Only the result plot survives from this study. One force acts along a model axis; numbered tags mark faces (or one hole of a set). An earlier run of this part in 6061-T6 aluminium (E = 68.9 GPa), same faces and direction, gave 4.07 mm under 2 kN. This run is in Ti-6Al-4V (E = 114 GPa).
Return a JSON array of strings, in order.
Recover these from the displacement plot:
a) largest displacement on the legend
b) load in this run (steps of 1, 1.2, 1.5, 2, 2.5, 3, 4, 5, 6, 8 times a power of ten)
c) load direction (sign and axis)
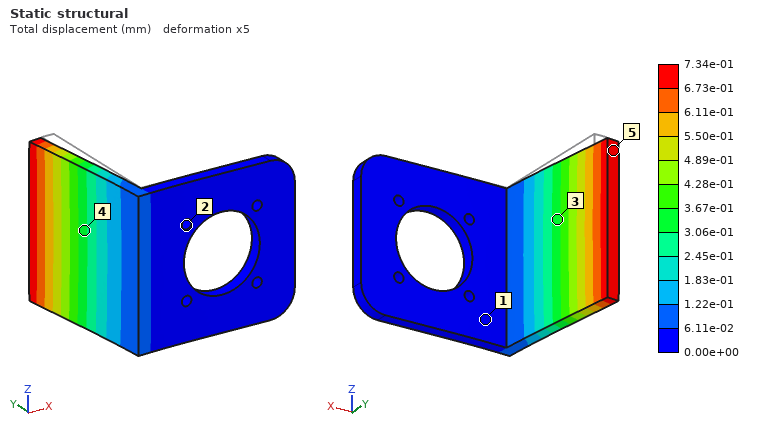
["7.34e-01 mm", "600 N", "-X"]
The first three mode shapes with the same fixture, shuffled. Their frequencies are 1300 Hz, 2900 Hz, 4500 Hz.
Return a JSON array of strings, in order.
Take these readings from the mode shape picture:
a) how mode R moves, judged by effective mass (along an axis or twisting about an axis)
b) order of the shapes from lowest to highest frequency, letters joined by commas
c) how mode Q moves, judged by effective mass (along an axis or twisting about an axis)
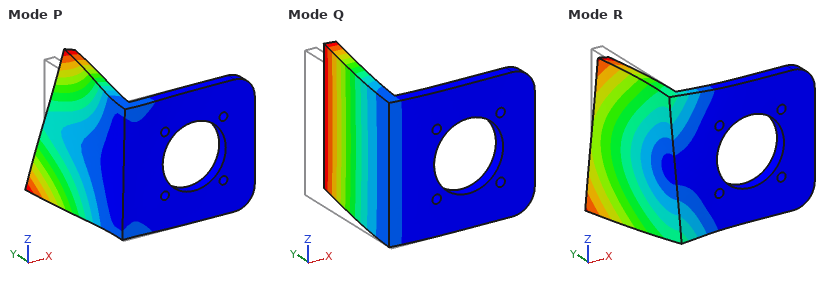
["along Z", "Q, R, P", "along X"]
